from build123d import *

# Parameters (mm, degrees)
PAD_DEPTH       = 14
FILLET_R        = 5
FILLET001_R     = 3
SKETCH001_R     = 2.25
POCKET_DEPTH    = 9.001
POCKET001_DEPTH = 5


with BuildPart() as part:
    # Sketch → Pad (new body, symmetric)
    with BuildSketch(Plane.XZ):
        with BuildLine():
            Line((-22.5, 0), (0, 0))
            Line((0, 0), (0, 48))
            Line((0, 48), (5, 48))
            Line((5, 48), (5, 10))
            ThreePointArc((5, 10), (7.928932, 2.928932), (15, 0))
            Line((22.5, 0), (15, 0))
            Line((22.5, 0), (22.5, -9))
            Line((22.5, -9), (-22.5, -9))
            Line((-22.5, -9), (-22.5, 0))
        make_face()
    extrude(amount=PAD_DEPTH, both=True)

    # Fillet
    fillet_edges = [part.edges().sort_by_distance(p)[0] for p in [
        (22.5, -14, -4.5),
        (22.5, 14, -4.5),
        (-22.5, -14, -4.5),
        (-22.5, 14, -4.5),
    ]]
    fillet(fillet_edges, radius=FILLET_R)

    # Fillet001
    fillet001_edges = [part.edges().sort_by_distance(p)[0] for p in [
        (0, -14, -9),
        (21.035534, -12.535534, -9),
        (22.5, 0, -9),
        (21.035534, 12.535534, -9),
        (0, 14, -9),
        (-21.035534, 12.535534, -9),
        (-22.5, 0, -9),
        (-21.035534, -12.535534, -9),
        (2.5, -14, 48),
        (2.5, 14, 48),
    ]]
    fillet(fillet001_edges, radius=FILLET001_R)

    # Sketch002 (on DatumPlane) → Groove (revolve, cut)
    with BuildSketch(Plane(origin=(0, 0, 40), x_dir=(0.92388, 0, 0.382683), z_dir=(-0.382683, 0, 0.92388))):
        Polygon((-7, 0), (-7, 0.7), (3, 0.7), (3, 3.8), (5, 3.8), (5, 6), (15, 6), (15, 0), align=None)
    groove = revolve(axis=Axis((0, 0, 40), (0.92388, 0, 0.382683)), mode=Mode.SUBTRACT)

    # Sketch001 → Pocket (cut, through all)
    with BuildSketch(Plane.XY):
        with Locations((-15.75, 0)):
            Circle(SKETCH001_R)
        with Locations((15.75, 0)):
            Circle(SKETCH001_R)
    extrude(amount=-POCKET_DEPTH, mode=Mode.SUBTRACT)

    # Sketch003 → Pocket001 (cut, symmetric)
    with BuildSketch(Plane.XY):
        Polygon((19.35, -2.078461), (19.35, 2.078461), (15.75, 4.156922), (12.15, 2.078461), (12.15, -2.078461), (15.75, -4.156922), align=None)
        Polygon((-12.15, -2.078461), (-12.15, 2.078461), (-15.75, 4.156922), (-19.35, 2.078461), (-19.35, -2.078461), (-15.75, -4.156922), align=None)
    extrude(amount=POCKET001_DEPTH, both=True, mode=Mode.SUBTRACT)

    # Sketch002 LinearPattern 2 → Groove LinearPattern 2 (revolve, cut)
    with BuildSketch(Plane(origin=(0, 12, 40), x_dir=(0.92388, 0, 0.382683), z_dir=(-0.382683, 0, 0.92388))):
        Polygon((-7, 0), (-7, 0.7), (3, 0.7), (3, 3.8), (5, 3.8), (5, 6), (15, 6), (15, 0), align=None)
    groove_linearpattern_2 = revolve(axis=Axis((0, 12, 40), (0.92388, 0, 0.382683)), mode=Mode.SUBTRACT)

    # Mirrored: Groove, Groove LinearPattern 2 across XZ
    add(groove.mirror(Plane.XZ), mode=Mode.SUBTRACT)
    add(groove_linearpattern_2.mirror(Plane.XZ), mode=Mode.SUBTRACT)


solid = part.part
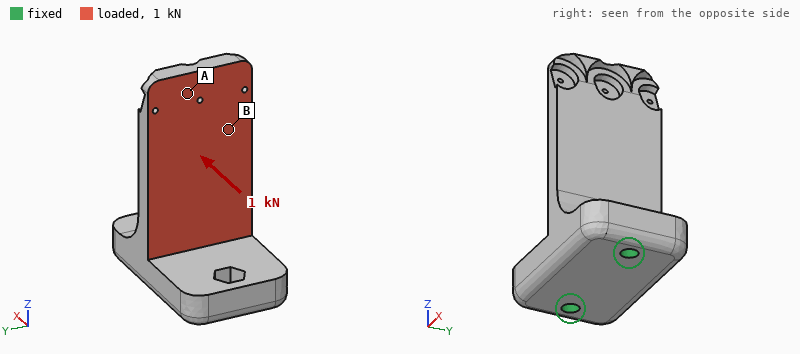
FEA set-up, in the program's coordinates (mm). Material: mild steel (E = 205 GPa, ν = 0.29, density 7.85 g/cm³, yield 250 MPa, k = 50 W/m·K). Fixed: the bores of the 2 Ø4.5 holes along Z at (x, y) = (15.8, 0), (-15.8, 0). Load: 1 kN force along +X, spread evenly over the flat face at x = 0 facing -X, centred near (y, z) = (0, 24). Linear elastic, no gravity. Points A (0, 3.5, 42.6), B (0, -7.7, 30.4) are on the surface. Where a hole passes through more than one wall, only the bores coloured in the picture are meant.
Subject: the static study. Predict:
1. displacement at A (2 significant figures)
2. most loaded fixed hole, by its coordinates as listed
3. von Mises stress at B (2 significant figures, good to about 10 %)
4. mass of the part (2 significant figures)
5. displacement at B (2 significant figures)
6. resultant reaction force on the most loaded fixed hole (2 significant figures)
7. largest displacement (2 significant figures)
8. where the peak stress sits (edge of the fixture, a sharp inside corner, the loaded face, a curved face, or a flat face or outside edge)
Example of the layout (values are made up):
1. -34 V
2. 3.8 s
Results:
1. 0.15 mm
2. (-15.8, 0)
3. 29 MPa
4. 130 g
5. 0.090 mm
6. 1.3 kN
7. 0.18 mm
8. a curved face
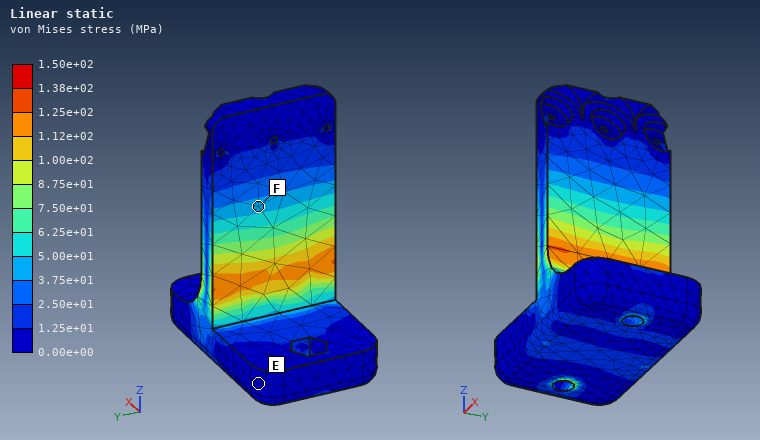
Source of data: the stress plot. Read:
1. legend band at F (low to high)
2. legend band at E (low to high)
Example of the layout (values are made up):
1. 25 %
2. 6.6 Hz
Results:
1. 3.75e+01 to 5.00e+01 MPa
2. 0.00e+00 to 1.25e+01 MPa
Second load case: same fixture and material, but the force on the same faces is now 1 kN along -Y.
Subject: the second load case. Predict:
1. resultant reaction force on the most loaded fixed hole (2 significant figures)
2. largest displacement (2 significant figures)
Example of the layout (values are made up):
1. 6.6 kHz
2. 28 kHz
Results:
1. 500 N
2. 86 µm
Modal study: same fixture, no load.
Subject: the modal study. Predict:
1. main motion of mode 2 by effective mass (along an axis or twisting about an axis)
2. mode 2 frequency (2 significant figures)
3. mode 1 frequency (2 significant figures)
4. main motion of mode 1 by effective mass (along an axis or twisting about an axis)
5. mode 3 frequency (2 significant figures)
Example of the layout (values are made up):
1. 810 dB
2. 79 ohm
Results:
1. along Y
2. 3000 Hz
3. 2300 Hz
4. along X
5. 7300 Hz
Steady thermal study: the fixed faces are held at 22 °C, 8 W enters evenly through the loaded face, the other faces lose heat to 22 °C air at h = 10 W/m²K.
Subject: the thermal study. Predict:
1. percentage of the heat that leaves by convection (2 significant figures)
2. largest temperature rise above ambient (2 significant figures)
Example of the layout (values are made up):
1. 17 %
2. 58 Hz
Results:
1. 7.8 %
2. 31 K
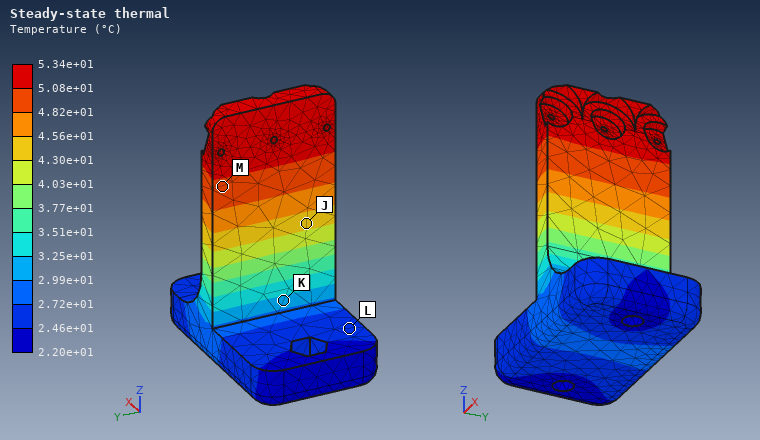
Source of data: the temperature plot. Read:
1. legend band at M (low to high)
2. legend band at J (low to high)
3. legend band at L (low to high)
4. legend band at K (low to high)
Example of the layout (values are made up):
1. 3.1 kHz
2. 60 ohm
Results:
1. 4.82e+01 to 5.08e+01 °C
2. 4.30e+01 to 4.56e+01 °C
3. 2.46e+01 to 2.72e+01 °C
4. 2.99e+01 to 3.25e+01 °C
